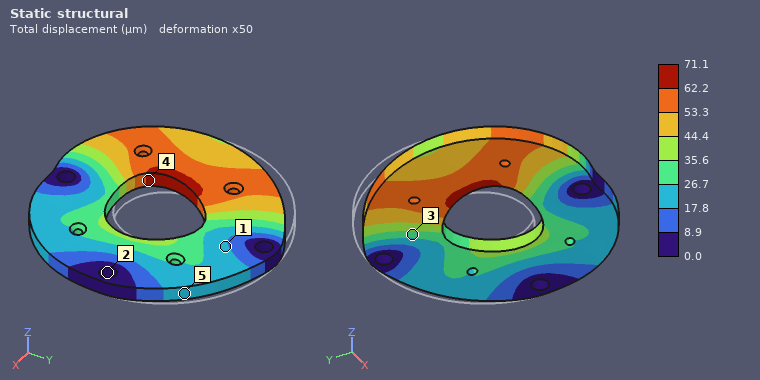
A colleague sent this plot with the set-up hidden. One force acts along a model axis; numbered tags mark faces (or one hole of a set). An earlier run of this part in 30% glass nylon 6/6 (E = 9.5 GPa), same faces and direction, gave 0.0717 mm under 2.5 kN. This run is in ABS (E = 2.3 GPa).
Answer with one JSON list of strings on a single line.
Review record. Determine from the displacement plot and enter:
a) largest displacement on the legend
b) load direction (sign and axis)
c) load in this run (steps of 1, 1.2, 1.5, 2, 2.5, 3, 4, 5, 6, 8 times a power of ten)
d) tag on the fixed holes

["71.1 µm", "-Y", "600 N", "2"]
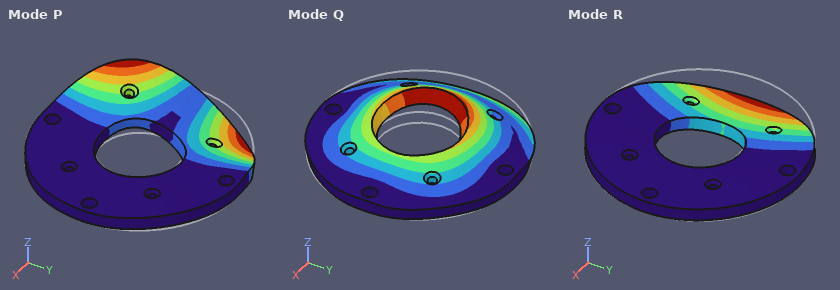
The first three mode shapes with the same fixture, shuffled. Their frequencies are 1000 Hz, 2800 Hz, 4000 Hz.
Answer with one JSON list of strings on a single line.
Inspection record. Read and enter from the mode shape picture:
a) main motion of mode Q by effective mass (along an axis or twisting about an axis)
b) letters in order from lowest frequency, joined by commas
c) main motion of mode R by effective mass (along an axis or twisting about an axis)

["along Z", "R, P, Q", "along Z"]
